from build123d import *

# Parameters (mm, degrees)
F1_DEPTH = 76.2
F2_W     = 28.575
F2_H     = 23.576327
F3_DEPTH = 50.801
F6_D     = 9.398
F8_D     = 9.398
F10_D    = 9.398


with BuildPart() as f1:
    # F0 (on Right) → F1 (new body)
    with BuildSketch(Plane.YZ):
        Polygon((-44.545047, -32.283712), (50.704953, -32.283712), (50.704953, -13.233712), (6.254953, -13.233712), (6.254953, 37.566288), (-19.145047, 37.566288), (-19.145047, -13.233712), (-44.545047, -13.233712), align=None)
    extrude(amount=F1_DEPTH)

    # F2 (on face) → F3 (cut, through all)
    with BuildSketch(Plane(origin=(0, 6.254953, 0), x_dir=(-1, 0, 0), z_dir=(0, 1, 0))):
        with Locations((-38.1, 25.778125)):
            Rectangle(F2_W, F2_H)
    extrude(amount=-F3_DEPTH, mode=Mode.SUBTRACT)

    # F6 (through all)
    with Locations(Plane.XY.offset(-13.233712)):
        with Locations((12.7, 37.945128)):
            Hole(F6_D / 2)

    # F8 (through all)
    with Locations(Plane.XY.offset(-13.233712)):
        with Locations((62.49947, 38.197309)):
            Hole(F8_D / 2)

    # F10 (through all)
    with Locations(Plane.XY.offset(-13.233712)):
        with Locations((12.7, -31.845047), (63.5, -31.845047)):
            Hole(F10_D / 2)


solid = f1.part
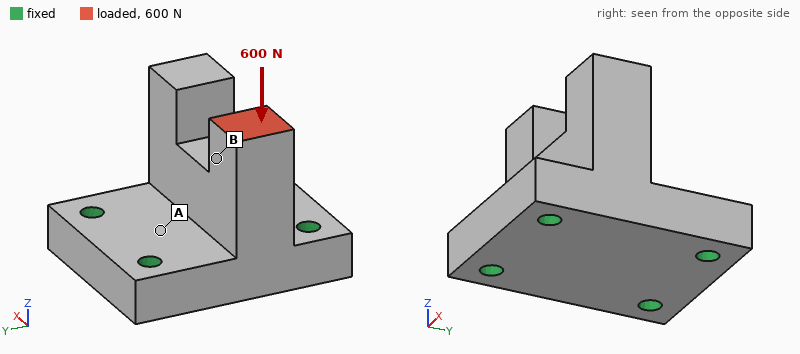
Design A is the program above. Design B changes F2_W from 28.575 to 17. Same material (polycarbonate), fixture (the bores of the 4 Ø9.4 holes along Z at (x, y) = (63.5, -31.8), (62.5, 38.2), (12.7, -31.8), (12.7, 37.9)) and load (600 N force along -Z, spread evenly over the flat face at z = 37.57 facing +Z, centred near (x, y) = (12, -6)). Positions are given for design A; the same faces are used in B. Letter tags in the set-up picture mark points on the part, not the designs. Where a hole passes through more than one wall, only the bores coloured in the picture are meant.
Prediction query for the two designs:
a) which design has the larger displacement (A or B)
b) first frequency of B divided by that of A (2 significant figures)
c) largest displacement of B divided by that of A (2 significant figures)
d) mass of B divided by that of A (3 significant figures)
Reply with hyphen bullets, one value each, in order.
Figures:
- A
- 0.94
- 0.86
- 1.03
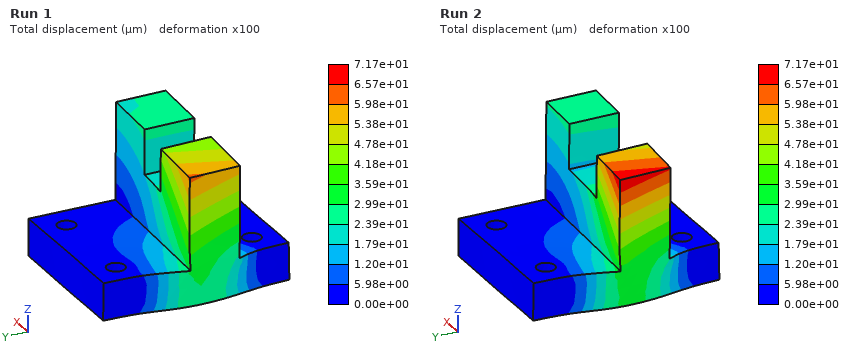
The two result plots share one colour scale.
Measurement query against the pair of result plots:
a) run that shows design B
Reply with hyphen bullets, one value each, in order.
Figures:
- Run 1
